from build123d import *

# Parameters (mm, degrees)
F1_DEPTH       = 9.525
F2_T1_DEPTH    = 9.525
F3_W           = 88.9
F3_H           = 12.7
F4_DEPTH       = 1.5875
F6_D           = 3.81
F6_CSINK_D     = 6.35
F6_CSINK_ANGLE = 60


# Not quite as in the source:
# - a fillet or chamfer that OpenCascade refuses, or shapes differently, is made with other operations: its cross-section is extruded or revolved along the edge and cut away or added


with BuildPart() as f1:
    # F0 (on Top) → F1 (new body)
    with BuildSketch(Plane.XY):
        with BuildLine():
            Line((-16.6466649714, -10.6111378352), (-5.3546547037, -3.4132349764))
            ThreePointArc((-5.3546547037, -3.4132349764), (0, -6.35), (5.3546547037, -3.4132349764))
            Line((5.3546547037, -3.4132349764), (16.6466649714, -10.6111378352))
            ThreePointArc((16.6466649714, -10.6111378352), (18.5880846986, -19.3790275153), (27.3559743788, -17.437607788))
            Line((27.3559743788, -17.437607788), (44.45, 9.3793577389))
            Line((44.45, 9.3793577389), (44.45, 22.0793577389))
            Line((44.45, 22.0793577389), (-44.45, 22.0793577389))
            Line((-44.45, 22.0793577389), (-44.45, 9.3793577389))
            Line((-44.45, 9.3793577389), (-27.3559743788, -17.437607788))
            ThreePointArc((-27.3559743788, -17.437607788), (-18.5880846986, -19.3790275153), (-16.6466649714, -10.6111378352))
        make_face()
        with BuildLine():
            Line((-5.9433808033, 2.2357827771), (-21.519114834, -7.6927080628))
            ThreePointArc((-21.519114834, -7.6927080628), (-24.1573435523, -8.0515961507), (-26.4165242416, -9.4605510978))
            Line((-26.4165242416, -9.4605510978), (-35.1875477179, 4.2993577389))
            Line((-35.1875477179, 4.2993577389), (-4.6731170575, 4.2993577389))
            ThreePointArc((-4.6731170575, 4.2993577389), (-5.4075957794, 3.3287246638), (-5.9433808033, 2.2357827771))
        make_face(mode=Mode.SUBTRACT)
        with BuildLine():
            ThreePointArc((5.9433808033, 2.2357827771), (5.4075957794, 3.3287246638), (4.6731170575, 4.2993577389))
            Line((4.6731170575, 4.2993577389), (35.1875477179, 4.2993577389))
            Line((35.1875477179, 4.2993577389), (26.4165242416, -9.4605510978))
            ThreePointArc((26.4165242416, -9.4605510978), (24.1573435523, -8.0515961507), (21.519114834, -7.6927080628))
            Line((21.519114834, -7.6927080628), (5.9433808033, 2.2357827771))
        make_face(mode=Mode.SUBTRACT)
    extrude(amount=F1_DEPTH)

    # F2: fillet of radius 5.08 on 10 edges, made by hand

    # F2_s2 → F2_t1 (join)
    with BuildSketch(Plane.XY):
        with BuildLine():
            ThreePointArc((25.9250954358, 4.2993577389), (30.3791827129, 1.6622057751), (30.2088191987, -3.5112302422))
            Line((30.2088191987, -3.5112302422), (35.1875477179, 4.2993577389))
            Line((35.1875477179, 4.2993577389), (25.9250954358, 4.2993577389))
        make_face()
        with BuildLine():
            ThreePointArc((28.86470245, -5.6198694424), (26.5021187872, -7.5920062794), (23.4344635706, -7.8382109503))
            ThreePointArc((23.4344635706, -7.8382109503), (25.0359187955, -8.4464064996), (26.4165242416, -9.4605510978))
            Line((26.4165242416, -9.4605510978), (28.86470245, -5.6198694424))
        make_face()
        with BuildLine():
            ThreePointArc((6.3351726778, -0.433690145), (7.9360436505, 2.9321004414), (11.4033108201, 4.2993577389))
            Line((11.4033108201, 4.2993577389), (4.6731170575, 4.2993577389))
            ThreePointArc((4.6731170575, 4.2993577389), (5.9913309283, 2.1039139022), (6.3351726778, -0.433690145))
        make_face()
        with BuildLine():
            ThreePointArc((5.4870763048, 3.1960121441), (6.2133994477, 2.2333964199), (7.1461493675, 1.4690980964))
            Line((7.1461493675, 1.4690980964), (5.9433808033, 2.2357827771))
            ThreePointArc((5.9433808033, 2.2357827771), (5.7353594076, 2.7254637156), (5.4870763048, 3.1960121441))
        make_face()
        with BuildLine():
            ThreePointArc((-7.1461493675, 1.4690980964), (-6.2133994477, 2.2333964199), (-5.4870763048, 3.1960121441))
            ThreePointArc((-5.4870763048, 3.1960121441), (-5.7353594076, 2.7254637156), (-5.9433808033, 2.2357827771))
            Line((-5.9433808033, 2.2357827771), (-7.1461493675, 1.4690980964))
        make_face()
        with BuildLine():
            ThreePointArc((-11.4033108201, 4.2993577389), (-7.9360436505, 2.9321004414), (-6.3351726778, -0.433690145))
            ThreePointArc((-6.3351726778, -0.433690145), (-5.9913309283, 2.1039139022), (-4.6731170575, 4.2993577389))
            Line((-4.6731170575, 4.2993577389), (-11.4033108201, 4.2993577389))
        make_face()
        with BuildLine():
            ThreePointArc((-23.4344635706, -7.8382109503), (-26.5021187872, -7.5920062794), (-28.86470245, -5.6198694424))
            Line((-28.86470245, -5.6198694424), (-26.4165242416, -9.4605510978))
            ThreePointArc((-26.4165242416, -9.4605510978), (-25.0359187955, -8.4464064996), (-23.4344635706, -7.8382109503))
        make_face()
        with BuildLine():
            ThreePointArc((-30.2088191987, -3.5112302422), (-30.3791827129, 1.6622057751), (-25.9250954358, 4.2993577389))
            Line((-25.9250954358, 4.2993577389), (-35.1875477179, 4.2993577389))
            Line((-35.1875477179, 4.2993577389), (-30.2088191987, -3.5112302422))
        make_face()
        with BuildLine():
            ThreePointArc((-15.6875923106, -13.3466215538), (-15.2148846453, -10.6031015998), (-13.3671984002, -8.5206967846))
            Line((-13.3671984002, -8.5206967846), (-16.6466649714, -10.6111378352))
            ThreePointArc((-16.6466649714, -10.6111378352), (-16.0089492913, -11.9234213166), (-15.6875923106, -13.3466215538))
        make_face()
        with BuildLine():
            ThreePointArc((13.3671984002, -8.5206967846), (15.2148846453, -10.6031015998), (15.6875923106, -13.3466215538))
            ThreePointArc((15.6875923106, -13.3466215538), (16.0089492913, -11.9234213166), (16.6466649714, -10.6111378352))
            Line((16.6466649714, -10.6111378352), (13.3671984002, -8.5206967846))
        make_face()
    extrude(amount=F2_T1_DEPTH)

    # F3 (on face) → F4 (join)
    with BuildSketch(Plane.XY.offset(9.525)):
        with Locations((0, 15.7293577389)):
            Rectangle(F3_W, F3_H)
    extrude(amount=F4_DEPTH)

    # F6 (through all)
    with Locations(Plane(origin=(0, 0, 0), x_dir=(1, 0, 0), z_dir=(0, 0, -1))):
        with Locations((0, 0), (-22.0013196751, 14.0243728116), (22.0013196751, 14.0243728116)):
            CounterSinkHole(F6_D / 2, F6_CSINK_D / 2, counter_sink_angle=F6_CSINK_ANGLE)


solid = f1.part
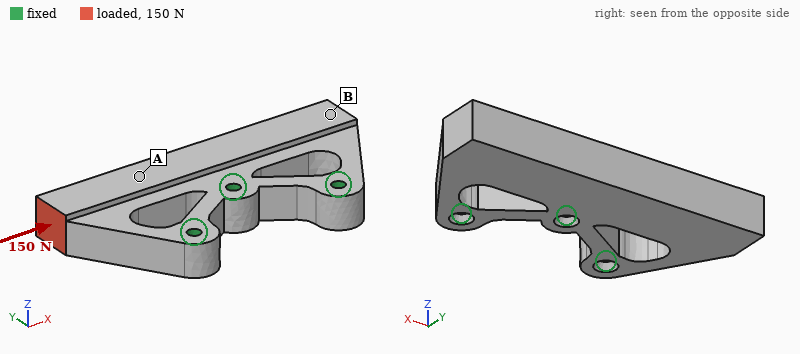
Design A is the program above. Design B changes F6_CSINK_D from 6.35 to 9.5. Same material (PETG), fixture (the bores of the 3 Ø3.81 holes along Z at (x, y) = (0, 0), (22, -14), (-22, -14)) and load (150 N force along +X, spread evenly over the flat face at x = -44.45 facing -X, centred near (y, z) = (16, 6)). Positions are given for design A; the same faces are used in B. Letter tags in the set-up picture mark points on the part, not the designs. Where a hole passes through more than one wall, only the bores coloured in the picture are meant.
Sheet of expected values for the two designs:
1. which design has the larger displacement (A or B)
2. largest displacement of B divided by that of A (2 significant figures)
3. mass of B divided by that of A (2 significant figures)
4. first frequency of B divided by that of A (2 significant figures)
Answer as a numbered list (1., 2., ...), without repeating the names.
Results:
1. B
2. 1.1
3. 0.99
4. 0.86
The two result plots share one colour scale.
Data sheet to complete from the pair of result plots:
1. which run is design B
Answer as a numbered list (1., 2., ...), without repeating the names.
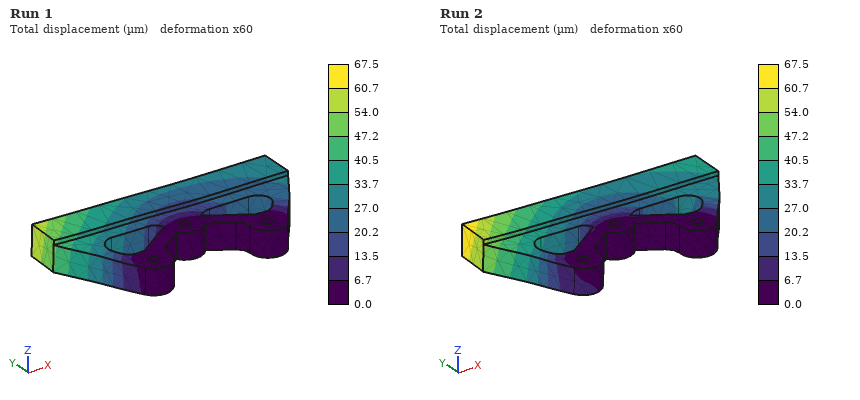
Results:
1. Run 2
